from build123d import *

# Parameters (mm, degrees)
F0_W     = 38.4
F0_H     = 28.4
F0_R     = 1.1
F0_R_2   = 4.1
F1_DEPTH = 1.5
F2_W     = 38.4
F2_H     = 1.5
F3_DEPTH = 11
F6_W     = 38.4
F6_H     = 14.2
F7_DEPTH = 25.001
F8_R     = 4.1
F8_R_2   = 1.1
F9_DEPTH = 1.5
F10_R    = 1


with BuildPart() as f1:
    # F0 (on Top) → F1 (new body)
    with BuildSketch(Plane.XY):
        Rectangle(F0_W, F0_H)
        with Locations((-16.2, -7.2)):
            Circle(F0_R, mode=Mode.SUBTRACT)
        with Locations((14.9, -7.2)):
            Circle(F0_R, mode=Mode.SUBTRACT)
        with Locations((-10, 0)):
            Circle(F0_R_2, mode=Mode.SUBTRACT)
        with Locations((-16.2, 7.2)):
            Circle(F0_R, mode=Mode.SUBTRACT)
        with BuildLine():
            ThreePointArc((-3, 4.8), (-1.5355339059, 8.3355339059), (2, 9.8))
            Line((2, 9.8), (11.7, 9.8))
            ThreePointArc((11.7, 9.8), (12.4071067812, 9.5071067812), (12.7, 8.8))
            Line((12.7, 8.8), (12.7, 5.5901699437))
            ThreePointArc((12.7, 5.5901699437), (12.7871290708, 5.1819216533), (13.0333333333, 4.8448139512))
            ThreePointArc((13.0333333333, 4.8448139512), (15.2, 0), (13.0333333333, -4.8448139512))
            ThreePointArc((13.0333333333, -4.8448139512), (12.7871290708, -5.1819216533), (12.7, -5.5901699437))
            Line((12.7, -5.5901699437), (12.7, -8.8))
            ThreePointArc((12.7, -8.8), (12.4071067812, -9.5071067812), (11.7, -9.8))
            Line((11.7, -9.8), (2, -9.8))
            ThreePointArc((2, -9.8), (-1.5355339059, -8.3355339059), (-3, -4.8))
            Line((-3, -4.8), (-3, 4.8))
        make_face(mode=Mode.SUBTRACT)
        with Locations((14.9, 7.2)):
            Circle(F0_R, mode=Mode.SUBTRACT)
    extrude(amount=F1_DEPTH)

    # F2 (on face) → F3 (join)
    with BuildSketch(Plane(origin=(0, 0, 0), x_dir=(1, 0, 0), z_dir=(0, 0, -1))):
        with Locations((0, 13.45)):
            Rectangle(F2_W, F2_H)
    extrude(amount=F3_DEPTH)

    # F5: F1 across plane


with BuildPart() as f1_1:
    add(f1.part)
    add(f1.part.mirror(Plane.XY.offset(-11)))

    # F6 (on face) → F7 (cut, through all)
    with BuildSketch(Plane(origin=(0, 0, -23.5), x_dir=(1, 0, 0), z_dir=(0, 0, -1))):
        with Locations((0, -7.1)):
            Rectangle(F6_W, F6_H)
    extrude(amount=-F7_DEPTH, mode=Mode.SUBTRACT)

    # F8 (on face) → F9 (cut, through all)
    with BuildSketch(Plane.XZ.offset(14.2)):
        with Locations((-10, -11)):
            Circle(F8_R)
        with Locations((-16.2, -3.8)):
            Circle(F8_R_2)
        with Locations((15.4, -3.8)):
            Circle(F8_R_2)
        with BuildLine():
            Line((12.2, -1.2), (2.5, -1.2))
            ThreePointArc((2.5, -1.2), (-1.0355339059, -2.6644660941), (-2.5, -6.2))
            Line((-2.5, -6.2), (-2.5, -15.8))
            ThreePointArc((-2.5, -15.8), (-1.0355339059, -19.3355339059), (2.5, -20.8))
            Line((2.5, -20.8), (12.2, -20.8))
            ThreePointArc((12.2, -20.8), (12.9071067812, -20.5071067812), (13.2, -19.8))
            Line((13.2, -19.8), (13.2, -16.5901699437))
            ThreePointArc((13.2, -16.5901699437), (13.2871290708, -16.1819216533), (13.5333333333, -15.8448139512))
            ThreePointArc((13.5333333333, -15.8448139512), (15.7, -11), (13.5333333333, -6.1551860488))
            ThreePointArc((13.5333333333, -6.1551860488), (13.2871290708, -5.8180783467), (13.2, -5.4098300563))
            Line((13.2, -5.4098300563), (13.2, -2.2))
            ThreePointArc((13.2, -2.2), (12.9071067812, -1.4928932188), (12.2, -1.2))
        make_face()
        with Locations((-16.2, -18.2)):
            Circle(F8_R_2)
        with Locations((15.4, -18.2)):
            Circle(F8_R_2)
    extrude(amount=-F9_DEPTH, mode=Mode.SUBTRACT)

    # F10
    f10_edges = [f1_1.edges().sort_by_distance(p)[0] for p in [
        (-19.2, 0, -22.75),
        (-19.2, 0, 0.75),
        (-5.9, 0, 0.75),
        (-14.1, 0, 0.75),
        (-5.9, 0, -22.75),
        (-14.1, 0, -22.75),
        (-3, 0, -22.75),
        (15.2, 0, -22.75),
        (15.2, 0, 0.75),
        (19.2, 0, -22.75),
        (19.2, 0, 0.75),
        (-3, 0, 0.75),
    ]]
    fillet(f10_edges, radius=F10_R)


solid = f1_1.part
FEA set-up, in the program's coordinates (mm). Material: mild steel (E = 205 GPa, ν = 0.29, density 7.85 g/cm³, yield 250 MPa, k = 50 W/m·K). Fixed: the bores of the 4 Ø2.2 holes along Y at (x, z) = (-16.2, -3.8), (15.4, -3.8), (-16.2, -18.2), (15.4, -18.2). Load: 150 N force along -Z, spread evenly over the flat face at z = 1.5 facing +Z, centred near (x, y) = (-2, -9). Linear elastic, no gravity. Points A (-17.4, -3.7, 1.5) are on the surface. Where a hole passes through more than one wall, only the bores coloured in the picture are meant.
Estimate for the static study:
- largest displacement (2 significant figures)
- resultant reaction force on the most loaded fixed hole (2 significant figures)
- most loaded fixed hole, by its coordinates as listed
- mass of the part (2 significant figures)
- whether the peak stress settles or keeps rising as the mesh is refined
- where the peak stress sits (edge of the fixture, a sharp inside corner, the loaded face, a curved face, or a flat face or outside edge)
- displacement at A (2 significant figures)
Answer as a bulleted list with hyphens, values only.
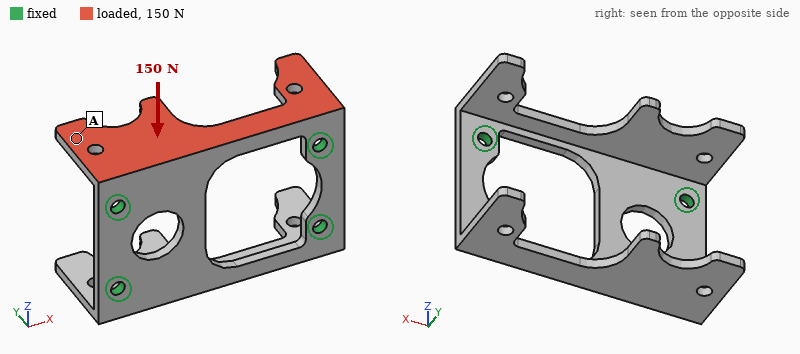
- 53 µm
- 75 N
- (-16.2, -3.8)
- 14 g
- keeps rising
- edge of the fixture
- 37 µm
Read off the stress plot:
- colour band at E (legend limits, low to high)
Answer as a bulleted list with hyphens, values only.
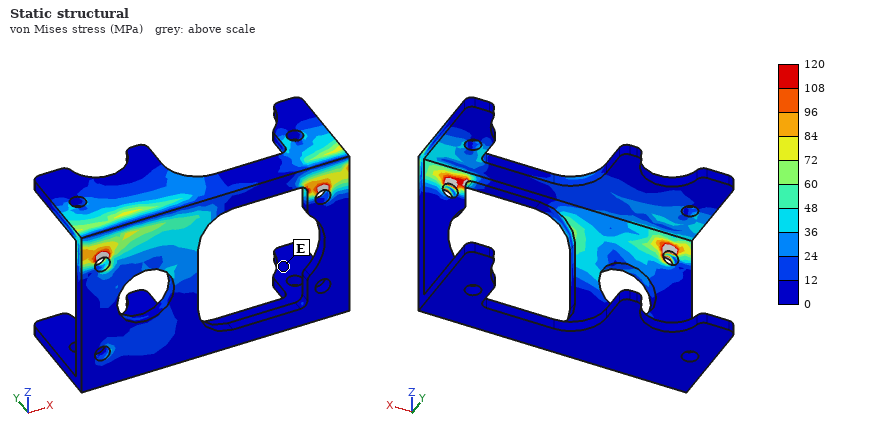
- 0 to 12 MPa
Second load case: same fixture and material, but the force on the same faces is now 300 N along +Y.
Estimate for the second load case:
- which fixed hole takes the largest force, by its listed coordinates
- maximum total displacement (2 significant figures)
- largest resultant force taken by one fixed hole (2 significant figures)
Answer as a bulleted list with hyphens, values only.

- (-16.2, -3.8)
- 56 µm
- 200 N
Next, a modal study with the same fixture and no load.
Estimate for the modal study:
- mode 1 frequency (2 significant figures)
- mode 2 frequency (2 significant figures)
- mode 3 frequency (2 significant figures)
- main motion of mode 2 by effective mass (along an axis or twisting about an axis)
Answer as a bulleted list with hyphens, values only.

- 5200 Hz
- 5400 Hz
- 6200 Hz
- along Z
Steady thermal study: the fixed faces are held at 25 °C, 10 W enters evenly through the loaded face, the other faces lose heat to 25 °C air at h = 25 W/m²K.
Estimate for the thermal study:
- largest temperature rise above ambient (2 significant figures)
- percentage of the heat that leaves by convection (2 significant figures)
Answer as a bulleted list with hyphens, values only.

- 63 K
- 9.9 %
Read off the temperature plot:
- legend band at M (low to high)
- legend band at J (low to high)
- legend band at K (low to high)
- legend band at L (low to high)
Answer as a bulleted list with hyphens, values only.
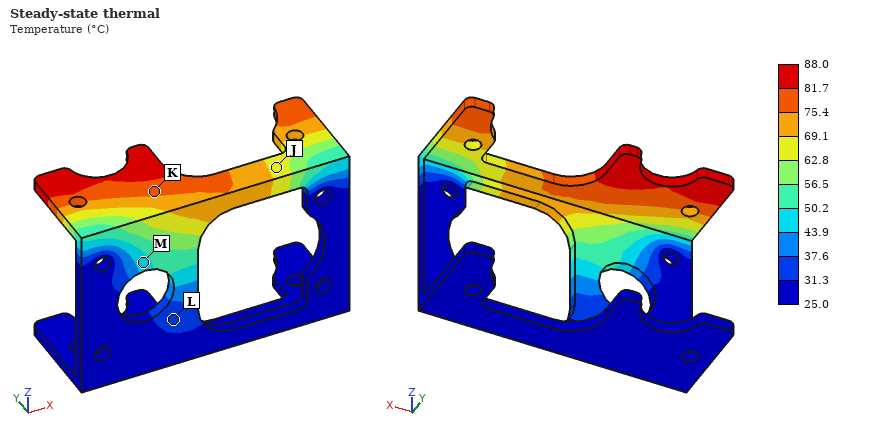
- 43.9 to 50.2 °C
- 62.8 to 69.1 °C
- 75.4 to 81.7 °C
- 31.3 to 37.6 °C
